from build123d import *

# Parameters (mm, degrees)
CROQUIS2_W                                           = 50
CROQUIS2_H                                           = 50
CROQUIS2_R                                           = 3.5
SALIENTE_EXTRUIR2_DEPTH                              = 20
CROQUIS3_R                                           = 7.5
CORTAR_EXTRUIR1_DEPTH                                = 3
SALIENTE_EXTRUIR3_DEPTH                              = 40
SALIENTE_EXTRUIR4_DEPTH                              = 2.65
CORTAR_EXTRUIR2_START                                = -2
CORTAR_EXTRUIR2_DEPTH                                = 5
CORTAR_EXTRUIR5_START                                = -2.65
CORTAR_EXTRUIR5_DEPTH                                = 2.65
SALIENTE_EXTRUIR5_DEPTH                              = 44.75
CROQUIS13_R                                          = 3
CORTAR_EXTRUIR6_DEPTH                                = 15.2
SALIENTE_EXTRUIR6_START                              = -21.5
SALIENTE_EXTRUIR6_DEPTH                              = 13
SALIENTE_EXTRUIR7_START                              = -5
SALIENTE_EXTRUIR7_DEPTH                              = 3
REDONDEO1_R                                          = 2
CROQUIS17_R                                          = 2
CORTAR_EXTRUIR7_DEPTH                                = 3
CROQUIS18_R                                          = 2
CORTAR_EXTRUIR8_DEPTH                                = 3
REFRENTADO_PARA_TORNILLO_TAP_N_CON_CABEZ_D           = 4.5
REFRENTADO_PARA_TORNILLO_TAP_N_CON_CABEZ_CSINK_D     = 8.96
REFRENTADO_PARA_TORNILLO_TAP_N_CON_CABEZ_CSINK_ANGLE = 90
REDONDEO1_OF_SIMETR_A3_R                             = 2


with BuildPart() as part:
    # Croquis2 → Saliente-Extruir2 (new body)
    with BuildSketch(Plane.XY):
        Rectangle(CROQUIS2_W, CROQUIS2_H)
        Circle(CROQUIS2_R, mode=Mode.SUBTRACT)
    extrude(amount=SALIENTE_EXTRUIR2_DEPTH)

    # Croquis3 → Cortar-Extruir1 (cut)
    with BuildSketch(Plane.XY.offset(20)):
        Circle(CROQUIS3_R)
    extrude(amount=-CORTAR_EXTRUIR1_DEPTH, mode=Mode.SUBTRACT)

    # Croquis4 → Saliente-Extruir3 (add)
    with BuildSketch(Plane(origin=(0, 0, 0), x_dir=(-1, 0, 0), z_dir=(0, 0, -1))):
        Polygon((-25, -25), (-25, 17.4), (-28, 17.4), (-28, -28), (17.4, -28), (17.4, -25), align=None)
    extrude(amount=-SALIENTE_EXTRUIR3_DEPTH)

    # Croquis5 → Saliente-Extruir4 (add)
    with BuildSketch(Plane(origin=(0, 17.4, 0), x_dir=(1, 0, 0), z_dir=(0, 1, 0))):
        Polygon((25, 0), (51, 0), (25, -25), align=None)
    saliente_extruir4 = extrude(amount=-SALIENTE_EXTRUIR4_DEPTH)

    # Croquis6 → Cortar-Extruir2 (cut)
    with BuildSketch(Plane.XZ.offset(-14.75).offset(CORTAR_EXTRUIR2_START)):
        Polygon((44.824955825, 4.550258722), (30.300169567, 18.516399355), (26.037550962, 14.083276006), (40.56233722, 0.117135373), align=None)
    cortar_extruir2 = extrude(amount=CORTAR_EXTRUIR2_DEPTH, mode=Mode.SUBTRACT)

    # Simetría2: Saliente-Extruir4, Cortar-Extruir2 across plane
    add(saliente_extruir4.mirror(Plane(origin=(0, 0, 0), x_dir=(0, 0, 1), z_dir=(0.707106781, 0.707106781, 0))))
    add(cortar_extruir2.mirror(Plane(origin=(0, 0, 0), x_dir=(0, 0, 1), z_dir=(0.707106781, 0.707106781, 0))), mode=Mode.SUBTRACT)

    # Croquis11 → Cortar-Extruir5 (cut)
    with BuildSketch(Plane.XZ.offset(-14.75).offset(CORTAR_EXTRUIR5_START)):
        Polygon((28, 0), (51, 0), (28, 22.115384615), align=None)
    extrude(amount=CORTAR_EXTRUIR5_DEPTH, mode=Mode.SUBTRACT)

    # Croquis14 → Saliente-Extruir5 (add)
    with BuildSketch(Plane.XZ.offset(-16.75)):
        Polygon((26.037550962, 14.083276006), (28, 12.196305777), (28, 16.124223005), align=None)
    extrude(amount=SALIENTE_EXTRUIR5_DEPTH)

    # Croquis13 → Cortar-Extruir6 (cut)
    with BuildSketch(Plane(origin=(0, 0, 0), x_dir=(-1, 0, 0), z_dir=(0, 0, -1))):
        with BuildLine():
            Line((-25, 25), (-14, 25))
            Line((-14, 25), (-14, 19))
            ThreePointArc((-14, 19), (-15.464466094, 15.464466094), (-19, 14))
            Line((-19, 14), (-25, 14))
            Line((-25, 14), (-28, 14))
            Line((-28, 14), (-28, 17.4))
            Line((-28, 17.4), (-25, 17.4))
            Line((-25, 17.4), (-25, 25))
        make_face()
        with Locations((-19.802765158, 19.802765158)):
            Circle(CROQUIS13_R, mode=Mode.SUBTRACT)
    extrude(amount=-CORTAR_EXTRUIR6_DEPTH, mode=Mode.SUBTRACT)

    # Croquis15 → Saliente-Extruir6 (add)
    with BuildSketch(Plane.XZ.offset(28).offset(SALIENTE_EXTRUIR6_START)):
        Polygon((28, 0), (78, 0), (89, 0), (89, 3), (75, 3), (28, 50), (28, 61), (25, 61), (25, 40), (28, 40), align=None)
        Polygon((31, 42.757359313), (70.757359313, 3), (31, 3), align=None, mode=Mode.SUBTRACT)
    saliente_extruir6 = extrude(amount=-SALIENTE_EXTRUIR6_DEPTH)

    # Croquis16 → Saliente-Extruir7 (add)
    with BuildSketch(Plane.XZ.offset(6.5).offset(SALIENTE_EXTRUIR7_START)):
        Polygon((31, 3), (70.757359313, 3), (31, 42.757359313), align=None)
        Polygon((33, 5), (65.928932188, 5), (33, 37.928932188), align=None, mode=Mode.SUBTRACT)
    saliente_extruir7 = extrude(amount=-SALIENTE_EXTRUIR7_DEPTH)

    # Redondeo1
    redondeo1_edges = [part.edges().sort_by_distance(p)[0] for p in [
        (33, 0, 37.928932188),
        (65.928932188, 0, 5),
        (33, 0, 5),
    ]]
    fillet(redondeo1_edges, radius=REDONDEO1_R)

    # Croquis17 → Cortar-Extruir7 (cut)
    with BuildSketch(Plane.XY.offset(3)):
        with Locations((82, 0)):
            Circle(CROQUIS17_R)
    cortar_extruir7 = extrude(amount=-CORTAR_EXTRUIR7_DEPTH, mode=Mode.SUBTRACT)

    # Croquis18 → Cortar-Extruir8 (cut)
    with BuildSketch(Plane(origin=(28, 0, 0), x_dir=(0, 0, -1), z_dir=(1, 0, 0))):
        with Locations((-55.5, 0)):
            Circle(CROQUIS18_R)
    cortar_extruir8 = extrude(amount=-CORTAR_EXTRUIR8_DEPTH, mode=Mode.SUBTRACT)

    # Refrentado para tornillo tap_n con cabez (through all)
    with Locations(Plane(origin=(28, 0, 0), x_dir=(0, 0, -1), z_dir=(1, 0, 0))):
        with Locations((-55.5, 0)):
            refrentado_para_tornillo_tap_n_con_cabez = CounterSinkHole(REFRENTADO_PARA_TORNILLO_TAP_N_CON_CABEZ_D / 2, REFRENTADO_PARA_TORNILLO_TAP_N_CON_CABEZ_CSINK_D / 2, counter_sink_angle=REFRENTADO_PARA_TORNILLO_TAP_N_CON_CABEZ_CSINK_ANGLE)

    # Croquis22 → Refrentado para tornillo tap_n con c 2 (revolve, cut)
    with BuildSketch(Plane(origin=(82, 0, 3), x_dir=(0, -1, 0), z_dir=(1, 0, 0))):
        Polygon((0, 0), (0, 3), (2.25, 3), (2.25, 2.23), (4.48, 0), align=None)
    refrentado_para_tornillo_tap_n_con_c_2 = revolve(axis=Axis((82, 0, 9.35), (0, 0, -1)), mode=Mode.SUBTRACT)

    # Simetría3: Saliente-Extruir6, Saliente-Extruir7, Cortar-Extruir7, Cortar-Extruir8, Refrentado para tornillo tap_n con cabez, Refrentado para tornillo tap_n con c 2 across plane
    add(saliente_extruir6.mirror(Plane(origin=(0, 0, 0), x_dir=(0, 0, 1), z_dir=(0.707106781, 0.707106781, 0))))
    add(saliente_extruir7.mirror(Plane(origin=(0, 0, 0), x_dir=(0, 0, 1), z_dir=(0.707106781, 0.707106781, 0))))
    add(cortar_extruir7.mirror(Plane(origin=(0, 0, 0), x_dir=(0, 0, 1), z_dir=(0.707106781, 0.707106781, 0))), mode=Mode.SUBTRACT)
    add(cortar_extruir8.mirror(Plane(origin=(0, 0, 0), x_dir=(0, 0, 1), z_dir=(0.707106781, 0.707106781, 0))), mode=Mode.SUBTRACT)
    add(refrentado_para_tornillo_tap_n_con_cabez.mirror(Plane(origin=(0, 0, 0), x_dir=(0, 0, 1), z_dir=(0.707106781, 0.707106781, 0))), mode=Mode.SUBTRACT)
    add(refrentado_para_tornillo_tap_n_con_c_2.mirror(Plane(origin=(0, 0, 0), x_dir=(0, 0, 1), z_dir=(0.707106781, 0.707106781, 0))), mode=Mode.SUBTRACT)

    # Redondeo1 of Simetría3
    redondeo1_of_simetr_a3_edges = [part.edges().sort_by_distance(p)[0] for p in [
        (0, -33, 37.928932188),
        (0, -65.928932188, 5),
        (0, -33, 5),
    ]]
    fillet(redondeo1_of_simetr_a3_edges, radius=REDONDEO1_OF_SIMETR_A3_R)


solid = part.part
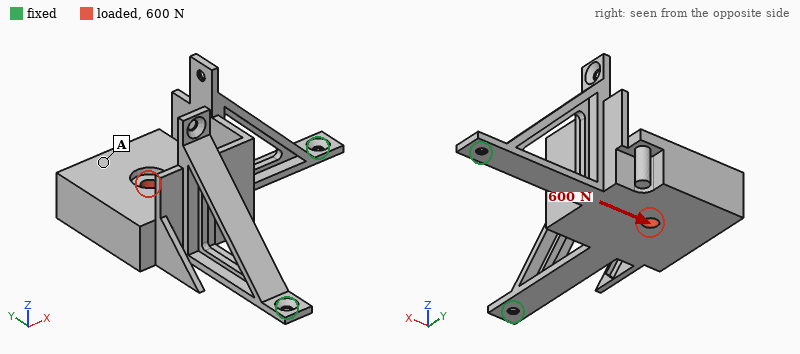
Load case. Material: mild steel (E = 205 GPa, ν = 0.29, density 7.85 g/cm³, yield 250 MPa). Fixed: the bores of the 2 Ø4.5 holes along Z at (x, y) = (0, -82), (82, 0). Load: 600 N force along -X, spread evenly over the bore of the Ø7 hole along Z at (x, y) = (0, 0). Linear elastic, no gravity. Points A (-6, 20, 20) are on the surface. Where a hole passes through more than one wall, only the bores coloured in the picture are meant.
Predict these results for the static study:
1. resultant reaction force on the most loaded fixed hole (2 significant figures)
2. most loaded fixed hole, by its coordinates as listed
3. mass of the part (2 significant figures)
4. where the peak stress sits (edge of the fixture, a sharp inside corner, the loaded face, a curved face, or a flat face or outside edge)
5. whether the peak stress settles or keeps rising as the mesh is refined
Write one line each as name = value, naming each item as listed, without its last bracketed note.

resultant reaction force on the most loaded fixed hole = 580 N
most loaded fixed hole, by its coordinates as listed = (82, 0)
mass of the part = 580 g
where the peak stress sits = edge of the fixture
whether the peak stress settles or keeps rising as the mesh is refined = keeps rising
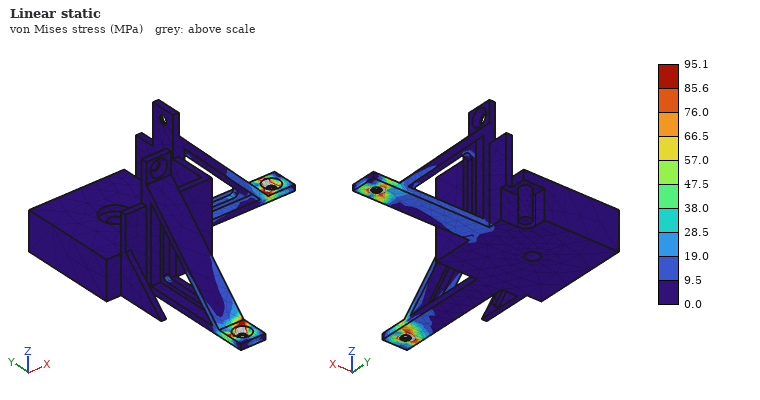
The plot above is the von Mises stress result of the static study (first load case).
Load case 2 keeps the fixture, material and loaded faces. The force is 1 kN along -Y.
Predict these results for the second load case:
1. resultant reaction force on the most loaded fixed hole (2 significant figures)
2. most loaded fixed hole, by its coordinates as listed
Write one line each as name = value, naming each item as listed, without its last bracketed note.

resultant reaction force on the most loaded fixed hole = 960 N
most loaded fixed hole, by its coordinates as listed = (0, -82)
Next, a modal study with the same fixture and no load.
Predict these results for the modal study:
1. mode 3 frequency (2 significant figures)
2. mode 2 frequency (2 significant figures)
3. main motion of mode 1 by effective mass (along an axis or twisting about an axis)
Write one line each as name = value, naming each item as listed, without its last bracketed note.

mode 3 frequency = 2100 Hz
mode 2 frequency = 1700 Hz
main motion of mode 1 by effective mass = along Z
